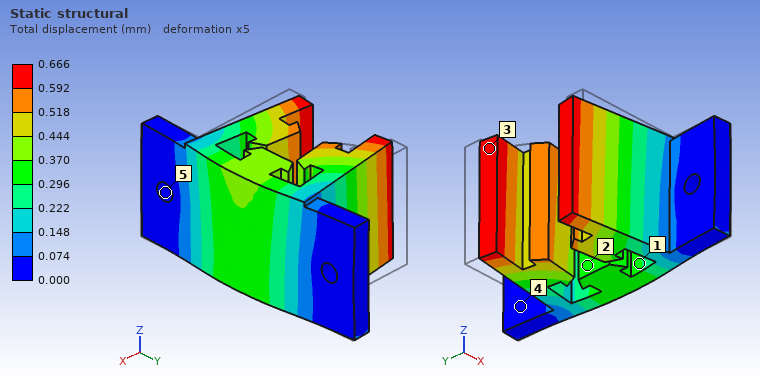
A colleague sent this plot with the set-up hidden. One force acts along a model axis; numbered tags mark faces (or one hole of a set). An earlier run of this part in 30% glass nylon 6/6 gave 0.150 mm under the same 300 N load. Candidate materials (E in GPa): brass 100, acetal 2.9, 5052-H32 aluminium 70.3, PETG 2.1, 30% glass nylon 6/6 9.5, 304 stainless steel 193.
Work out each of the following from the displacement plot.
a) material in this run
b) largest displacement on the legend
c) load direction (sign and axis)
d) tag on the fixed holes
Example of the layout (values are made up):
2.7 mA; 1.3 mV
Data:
PETG; 0.666 mm; +X; 5
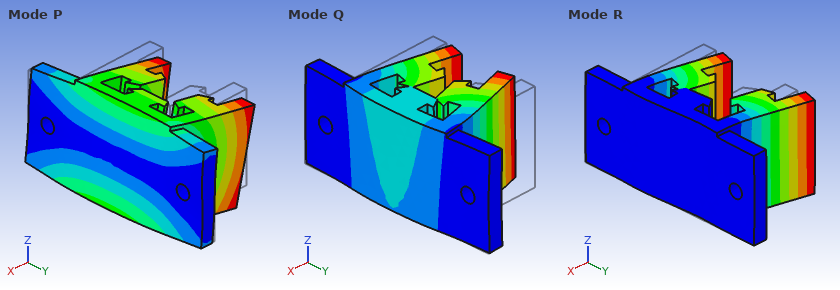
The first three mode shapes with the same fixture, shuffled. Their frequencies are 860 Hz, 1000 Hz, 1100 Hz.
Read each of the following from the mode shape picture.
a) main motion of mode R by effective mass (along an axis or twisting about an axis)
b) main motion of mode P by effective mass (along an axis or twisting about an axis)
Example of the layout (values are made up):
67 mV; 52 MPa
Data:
along Y; along Z
